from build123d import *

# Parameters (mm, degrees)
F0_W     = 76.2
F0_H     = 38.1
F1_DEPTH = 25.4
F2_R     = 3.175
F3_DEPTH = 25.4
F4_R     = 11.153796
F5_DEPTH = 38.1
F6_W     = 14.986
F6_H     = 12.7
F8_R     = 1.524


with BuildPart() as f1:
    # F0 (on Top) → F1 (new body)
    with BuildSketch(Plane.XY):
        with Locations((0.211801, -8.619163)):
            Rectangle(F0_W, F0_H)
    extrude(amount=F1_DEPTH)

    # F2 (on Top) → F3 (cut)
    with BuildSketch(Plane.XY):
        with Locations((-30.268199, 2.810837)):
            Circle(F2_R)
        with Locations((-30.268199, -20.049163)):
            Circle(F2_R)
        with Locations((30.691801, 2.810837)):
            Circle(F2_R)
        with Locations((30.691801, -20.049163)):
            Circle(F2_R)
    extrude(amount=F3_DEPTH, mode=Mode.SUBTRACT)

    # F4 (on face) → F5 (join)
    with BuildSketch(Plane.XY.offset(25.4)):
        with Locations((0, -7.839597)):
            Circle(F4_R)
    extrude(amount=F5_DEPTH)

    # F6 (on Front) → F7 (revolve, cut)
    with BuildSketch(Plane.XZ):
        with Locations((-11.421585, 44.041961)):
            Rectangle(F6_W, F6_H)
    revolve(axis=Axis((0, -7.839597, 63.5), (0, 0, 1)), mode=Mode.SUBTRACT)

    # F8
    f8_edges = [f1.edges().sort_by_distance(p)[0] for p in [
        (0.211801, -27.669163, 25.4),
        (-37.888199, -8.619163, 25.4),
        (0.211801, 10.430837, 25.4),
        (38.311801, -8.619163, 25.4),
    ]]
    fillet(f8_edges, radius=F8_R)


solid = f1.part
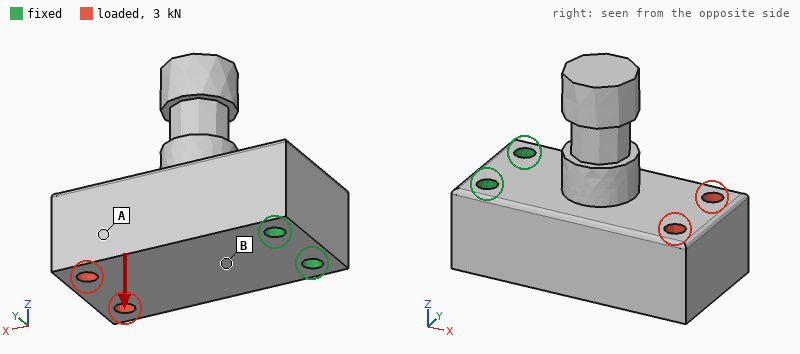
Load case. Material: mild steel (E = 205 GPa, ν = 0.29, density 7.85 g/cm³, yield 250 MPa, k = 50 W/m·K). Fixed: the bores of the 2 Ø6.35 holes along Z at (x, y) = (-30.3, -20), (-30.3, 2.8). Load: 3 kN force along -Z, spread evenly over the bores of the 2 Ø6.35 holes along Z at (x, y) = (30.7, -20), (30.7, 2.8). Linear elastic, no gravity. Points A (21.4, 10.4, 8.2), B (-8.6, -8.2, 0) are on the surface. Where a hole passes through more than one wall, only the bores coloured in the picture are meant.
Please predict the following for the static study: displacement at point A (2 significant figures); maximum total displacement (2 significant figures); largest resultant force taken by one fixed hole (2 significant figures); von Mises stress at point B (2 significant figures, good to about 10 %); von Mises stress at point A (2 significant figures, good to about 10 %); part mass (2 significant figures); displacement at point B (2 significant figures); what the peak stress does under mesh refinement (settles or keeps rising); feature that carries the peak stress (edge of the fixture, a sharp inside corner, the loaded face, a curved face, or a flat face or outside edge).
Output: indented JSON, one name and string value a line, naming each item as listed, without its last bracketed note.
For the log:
{
  "displacement at point A": "18 µm",
  "maximum total displacement": "28 µm",
  "largest resultant force taken by one fixed hole": "1.5 kN",
  "von Mises stress at point B": "27 MPa",
  "von Mises stress at point A": "8.8 MPa",
  "part mass": "650 g",
  "displacement at point B": "6.3 µm",
  "what the peak stress does under mesh refinement": "keeps rising",
  "feature that carries the peak stress": "edge of the fixture"
}
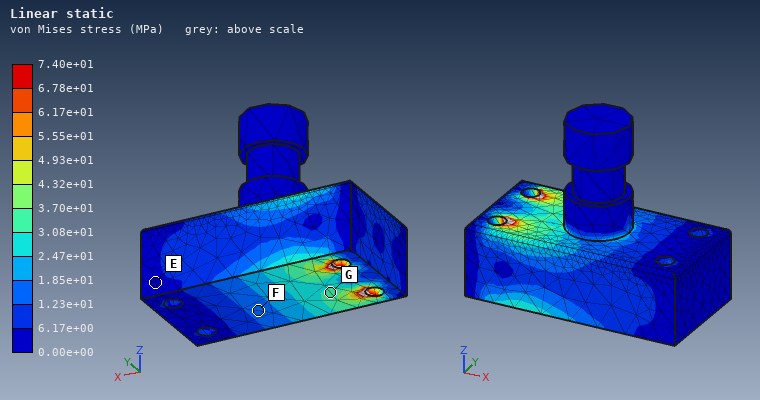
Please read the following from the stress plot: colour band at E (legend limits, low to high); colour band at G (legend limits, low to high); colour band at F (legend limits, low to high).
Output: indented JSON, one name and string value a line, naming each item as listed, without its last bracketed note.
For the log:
{
  "colour band at E": "0.00e+00 to 6.17e+00 MPa",
  "colour band at G": "3.08e+01 to 3.70e+01 MPa",
  "colour band at F": "1.23e+01 to 1.85e+01 MPa"
}
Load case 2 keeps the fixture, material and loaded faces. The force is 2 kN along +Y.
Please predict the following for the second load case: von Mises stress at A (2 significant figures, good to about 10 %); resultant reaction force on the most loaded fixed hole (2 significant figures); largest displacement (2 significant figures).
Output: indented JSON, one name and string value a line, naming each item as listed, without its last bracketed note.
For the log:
{
  "von Mises stress at A": "3.5 MPa",
  "resultant reaction force on the most loaded fixed hole": "4.7 kN",
  "largest displacement": "9.9 µm"
}
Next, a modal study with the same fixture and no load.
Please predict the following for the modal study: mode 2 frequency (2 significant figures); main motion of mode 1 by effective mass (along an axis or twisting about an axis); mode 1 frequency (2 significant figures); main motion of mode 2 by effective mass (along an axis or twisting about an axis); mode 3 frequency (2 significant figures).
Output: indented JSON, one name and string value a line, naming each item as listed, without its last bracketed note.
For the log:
{
  "mode 2 frequency": "5100 Hz",
  "main motion of mode 1 by effective mass": "along Z",
  "mode 1 frequency": "3600 Hz",
  "main motion of mode 2 by effective mass": "along Y",
  "mode 3 frequency": "6100 Hz"
}
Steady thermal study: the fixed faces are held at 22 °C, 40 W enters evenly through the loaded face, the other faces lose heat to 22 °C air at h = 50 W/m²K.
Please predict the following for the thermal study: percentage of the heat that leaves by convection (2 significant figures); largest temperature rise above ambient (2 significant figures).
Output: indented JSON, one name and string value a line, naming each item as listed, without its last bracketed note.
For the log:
{
  "percentage of the heat that leaves by convection": "31 %",
  "largest temperature rise above ambient": "41 K"
}
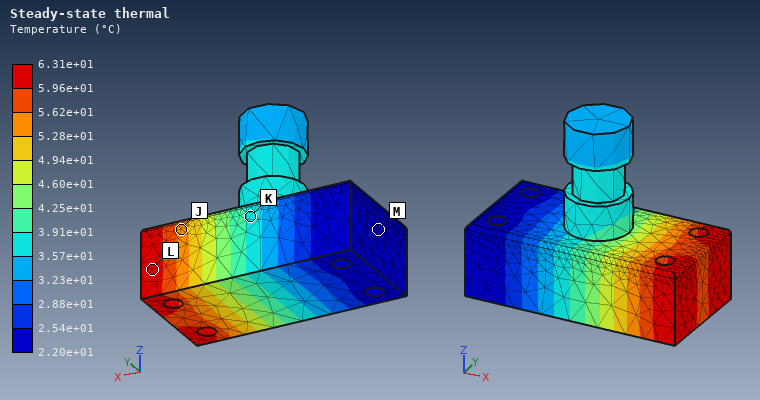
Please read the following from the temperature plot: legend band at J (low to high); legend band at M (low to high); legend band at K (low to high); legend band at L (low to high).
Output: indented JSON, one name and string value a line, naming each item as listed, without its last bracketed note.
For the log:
{
  "legend band at J": "5.28e+01 to 5.62e+01 °C",
  "legend band at M": "2.20e+01 to 2.54e+01 °C",
  "legend band at K": "3.57e+01 to 3.91e+01 °C",
  "legend band at L": "5.96e+01 to 6.31e+01 °C"
}
